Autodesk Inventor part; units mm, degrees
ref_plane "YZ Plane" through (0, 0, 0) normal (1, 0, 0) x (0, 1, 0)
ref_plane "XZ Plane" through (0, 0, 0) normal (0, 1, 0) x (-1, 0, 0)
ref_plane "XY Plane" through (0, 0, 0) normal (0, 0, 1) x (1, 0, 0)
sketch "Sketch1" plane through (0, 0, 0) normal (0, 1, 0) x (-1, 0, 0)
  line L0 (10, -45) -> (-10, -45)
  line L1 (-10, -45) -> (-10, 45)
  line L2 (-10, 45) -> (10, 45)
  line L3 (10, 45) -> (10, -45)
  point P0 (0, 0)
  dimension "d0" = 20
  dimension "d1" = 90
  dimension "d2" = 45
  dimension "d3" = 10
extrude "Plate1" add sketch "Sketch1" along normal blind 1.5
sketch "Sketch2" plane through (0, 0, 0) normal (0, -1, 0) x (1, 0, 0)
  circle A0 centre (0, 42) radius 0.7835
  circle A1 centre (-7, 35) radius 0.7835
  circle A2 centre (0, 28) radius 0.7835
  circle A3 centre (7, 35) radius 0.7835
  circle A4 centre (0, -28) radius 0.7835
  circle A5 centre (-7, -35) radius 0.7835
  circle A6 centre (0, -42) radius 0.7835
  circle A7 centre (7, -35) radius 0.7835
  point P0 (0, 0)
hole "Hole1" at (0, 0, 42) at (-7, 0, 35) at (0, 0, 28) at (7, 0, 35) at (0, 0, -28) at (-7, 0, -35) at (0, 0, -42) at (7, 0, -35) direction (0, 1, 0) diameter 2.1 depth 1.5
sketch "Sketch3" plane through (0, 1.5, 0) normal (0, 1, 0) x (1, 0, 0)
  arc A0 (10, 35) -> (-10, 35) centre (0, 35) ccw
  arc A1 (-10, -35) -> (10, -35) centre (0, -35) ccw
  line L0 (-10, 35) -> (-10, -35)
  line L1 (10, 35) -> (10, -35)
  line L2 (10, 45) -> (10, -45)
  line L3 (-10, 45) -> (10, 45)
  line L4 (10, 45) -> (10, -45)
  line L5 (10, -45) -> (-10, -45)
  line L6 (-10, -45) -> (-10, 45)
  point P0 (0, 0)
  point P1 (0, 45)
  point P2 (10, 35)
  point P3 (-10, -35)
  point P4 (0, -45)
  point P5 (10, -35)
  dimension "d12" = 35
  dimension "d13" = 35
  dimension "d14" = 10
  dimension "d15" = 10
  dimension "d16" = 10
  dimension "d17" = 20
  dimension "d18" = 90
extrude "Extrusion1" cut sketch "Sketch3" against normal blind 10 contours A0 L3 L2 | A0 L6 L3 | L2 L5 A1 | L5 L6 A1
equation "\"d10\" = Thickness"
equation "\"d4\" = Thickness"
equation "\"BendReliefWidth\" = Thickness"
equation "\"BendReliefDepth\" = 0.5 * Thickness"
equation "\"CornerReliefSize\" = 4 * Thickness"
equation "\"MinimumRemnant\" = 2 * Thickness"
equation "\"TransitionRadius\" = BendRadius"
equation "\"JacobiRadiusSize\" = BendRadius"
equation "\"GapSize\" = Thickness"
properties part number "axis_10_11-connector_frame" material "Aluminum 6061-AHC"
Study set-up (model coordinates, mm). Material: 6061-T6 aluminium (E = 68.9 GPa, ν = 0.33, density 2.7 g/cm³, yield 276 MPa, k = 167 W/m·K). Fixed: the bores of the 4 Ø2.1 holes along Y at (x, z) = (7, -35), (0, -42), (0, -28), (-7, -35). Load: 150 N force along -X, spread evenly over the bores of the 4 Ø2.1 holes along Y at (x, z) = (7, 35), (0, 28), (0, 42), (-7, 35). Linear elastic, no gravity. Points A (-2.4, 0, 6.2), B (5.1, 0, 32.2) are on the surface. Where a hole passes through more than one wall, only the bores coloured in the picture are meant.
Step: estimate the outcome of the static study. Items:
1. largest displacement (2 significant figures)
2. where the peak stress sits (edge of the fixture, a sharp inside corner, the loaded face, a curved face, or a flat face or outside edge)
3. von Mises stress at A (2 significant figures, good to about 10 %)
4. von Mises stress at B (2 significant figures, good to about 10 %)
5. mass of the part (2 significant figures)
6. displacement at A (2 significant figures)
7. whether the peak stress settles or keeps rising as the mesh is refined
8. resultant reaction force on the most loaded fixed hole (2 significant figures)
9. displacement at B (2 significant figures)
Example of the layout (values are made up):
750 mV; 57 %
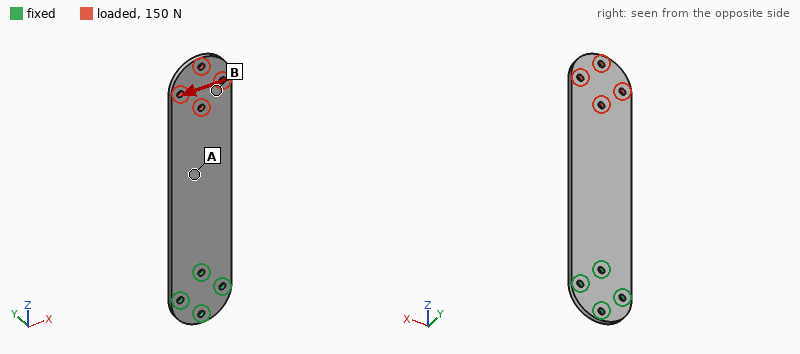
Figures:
0.31 mm; edge of the fixture; 16 MPa; 8.9 MPa; 6.8 g; 0.11 mm; keeps rising; 500 N; 0.24 mm
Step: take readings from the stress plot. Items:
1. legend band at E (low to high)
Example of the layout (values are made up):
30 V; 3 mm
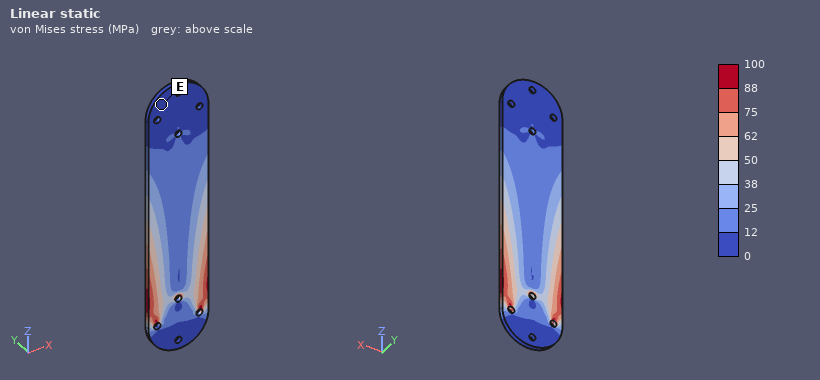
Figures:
0 to 12 MPa
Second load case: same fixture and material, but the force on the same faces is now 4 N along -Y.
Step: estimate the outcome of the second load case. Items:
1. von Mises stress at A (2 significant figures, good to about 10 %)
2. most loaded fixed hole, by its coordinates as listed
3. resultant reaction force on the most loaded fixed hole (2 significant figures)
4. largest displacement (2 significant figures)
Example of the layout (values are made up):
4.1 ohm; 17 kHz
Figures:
15 MPa; (0, -28); 24 N; 1.1 mm
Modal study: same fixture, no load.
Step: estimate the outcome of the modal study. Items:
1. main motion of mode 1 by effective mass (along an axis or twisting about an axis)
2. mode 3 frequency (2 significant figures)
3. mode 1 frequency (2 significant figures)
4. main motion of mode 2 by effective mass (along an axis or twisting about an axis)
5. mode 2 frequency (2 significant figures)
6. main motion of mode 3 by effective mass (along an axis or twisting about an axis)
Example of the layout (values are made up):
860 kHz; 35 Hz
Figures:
along Y; 1700 Hz; 250 Hz; along Y; 1500 Hz; twisting about Z
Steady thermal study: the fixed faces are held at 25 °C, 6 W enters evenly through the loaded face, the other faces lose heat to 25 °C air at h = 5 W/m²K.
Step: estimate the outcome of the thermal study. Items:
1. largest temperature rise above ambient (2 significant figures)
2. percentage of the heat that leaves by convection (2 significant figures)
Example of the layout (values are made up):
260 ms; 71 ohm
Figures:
75 K; 10 %
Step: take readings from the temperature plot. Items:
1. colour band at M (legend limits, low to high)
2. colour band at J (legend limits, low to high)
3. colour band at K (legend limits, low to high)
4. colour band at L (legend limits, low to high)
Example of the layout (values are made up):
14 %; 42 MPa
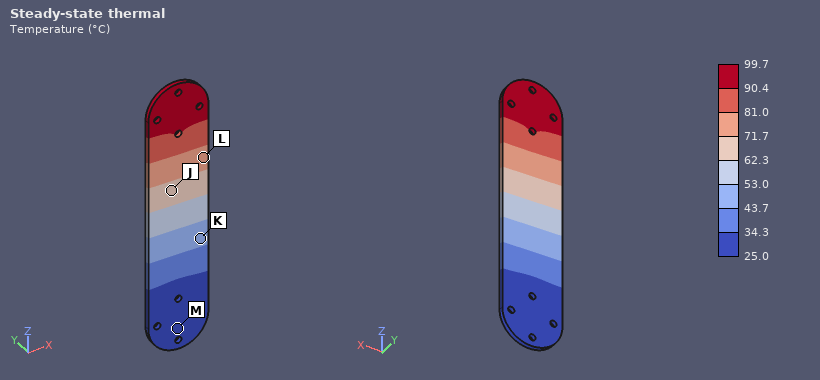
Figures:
25.0 to 34.3 °C; 62.3 to 71.7 °C; 43.7 to 53.0 °C; 71.7 to 81.0 °C
